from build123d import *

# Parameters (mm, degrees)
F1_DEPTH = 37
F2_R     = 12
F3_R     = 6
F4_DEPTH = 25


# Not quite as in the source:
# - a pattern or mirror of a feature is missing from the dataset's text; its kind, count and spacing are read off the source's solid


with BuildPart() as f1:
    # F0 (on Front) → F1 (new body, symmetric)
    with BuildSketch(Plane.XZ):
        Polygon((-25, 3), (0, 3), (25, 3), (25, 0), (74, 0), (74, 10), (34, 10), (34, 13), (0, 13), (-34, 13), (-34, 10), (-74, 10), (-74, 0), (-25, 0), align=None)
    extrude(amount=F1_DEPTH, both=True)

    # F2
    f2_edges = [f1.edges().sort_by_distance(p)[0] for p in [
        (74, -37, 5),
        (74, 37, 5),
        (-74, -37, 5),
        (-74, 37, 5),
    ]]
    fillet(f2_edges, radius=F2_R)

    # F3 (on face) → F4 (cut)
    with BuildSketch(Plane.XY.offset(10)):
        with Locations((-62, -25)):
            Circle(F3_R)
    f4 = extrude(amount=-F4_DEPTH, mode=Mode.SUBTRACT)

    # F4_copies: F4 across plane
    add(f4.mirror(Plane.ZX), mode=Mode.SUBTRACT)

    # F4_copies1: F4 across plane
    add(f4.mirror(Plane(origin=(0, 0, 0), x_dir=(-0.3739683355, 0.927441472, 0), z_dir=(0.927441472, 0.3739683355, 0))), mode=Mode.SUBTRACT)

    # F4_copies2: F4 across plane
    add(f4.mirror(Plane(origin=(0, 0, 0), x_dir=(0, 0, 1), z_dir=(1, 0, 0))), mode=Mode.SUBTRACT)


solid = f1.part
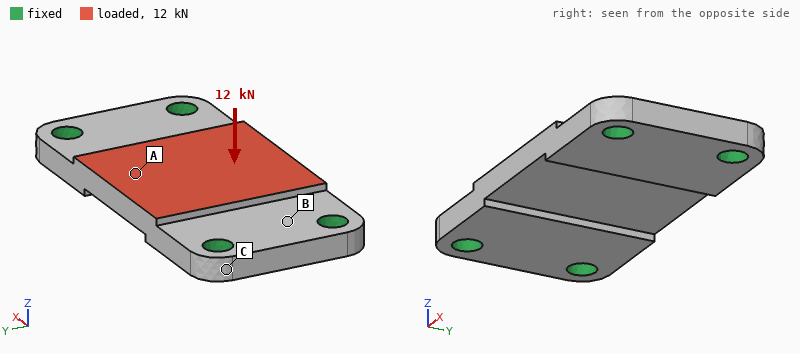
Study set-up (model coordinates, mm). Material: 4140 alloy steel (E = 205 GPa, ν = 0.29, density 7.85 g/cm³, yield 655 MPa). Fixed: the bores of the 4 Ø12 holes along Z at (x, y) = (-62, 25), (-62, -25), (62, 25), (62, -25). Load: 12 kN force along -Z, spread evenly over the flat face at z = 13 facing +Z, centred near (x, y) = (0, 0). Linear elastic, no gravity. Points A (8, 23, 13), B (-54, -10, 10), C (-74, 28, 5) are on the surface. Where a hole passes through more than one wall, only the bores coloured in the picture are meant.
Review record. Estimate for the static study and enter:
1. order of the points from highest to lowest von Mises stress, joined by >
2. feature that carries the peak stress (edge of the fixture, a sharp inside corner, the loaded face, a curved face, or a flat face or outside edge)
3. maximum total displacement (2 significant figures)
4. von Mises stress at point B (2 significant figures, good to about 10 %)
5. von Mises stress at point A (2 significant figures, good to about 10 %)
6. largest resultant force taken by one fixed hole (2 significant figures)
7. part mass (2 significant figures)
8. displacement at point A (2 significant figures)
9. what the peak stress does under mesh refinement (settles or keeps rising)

A > B > C
edge of the fixture
61 µm
42 MPa
71 MPa
5.7 kN
850 g
56 µm
keeps rising
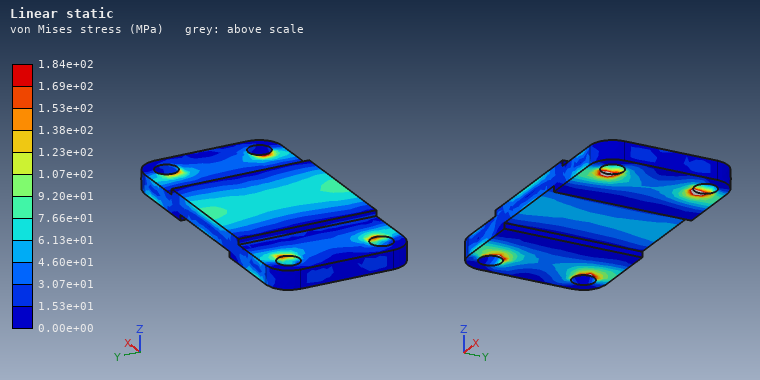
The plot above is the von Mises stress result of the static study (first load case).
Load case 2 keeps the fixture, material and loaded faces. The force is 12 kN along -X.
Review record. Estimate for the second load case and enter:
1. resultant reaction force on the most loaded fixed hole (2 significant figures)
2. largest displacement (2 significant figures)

3.1 kN
2.4 µm
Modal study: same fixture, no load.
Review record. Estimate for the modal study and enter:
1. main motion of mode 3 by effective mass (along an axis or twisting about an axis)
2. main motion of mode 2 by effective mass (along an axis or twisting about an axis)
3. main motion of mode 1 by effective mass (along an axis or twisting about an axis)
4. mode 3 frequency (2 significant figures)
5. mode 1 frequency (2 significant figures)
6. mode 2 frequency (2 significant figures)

twisting about Y
twisting about X
along Z
9000 Hz
3700 Hz
5400 Hz
